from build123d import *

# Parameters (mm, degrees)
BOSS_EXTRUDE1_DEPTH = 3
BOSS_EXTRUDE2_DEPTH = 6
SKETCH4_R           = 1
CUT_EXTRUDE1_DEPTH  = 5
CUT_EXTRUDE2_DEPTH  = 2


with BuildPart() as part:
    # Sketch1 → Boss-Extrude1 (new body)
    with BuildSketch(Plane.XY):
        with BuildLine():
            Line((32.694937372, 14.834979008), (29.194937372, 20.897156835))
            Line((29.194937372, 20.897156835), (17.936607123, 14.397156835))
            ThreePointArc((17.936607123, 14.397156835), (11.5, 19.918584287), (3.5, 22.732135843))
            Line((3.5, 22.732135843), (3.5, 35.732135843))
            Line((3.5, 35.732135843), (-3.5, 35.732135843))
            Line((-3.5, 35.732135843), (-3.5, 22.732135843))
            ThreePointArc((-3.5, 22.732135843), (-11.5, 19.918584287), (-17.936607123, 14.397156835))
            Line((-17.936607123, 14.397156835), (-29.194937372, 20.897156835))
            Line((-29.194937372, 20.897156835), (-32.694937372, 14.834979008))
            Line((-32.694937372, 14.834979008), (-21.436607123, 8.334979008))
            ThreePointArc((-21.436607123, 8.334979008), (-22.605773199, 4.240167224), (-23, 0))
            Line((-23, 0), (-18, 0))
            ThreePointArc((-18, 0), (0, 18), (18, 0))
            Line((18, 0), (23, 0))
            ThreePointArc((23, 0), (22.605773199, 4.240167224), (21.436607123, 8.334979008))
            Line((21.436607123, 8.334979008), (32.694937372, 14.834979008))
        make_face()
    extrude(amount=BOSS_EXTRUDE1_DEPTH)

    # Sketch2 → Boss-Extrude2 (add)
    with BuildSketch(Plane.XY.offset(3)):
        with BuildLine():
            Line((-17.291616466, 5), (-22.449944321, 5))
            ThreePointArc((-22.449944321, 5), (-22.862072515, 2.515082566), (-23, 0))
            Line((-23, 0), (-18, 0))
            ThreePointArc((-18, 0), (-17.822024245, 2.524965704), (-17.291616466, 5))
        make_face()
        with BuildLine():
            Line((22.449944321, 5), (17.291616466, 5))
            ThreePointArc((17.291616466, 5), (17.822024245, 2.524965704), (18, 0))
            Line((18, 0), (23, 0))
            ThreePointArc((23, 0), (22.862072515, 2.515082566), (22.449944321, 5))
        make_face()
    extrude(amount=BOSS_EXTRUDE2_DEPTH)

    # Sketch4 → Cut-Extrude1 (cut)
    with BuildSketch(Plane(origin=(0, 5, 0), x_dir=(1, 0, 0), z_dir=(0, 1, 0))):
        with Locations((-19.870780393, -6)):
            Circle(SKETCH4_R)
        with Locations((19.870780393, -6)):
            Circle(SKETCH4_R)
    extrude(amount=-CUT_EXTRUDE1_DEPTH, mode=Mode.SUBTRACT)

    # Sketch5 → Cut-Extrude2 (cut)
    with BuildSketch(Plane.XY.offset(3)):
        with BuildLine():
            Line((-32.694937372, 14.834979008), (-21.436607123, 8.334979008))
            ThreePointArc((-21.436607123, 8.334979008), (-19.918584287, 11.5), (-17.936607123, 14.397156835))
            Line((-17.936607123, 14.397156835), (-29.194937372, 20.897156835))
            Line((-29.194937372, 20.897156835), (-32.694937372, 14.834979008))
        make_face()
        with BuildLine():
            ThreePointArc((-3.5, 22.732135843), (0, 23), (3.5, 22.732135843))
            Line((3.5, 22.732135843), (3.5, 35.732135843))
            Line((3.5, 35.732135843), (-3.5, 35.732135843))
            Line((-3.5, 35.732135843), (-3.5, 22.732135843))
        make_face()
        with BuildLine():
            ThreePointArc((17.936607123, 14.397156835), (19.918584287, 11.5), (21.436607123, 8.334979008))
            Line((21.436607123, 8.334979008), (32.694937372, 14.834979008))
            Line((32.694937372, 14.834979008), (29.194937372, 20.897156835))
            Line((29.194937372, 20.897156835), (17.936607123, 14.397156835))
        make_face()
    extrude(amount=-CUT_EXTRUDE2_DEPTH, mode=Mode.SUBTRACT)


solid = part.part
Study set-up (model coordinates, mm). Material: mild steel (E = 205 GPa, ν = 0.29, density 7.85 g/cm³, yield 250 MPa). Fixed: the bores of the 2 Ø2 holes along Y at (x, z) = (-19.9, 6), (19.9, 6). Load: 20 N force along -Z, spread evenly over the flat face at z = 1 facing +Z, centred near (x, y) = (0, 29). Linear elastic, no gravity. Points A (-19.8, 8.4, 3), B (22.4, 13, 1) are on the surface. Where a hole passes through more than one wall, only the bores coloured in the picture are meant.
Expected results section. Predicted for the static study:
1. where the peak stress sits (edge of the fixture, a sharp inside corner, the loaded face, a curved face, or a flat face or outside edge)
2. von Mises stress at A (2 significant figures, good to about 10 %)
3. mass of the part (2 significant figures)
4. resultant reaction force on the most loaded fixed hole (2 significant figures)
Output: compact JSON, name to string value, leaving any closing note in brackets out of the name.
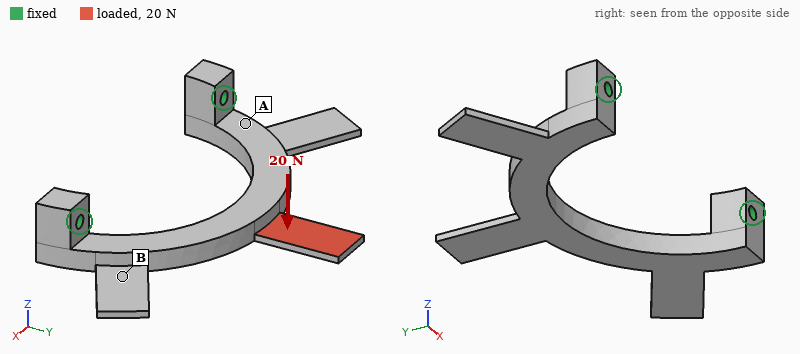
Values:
{"where the peak stress sits": "a flat face or outside edge", "von Mises stress at A": "29 MPa", "mass of the part": "12 g", "resultant reaction force on the most loaded fixed hole": "10 N"}
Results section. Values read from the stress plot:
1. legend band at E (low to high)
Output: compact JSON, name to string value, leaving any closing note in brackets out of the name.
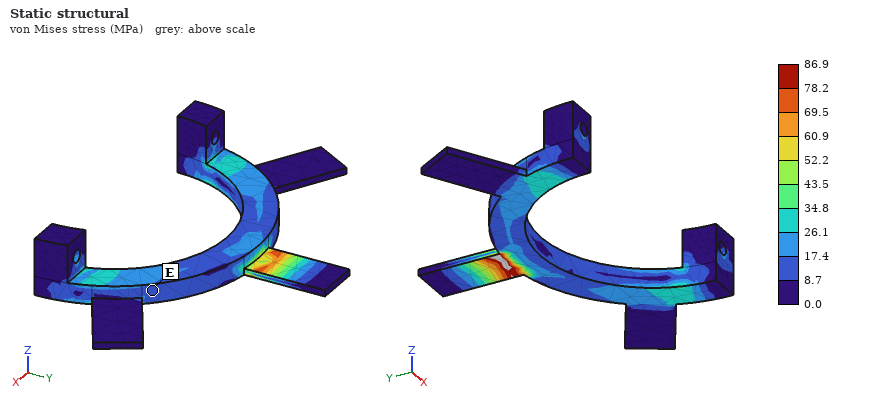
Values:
{"legend band at E": "8.7 to 17.4 MPa"}
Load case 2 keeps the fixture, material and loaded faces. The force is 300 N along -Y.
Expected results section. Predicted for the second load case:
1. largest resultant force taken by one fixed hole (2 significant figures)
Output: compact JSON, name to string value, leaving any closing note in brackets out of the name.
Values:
{"largest resultant force taken by one fixed hole": "200 N"}
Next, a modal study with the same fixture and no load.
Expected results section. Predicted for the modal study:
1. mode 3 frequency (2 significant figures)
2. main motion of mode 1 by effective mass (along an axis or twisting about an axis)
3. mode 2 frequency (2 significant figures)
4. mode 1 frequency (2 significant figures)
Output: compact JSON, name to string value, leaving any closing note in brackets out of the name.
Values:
{"mode 3 frequency": "4400 Hz", "main motion of mode 1 by effective mass": "along Z", "mode 2 frequency": "4400 Hz", "mode 1 frequency": "2700 Hz"}
